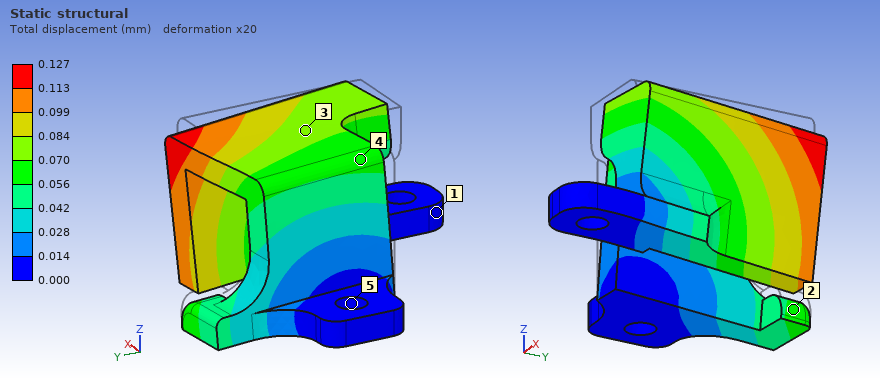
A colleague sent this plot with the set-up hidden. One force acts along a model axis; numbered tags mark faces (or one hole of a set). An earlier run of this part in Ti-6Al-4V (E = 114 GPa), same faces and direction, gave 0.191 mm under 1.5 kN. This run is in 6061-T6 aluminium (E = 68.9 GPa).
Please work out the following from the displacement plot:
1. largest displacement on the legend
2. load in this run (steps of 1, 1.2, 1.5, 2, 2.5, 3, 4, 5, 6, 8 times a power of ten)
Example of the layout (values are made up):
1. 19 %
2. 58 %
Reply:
1. 0.127 mm
2. 600 N
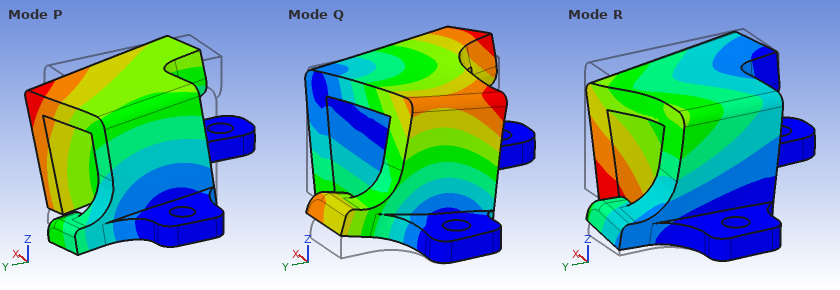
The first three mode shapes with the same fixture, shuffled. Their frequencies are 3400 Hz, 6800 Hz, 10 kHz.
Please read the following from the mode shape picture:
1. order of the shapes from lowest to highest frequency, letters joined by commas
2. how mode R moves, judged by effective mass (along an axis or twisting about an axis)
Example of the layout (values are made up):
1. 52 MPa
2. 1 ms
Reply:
1. P, R, Q
2. along X
